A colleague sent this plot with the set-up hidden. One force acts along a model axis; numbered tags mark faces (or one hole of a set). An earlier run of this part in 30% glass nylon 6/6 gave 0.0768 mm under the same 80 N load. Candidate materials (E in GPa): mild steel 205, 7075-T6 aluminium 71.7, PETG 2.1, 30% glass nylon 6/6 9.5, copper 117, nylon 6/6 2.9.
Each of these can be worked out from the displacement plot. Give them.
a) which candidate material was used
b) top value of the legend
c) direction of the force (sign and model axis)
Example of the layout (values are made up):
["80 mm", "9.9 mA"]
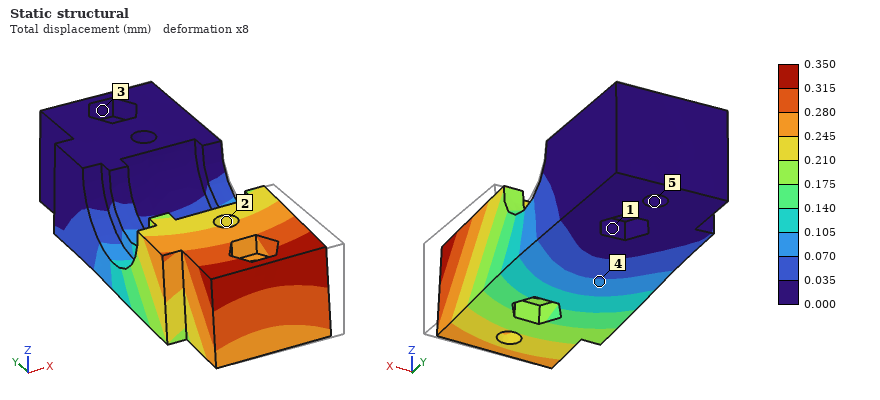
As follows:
["PETG", "0.350 mm", "-X"]
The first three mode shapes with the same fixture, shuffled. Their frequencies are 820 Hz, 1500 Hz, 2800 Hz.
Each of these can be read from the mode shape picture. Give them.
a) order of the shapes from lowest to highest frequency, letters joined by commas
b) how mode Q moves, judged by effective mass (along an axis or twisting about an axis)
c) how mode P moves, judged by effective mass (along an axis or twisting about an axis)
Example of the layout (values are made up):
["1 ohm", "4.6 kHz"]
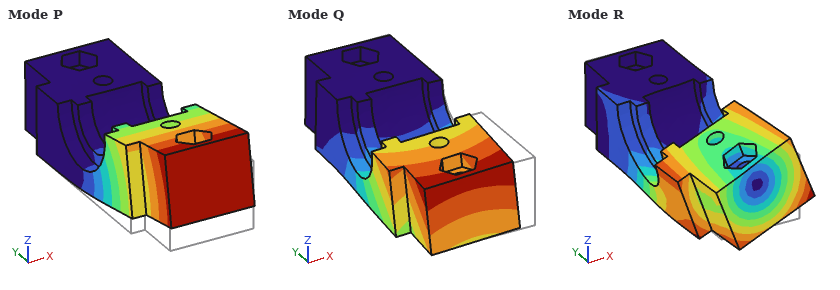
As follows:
["P, Q, R", "along X", "along Z"]
